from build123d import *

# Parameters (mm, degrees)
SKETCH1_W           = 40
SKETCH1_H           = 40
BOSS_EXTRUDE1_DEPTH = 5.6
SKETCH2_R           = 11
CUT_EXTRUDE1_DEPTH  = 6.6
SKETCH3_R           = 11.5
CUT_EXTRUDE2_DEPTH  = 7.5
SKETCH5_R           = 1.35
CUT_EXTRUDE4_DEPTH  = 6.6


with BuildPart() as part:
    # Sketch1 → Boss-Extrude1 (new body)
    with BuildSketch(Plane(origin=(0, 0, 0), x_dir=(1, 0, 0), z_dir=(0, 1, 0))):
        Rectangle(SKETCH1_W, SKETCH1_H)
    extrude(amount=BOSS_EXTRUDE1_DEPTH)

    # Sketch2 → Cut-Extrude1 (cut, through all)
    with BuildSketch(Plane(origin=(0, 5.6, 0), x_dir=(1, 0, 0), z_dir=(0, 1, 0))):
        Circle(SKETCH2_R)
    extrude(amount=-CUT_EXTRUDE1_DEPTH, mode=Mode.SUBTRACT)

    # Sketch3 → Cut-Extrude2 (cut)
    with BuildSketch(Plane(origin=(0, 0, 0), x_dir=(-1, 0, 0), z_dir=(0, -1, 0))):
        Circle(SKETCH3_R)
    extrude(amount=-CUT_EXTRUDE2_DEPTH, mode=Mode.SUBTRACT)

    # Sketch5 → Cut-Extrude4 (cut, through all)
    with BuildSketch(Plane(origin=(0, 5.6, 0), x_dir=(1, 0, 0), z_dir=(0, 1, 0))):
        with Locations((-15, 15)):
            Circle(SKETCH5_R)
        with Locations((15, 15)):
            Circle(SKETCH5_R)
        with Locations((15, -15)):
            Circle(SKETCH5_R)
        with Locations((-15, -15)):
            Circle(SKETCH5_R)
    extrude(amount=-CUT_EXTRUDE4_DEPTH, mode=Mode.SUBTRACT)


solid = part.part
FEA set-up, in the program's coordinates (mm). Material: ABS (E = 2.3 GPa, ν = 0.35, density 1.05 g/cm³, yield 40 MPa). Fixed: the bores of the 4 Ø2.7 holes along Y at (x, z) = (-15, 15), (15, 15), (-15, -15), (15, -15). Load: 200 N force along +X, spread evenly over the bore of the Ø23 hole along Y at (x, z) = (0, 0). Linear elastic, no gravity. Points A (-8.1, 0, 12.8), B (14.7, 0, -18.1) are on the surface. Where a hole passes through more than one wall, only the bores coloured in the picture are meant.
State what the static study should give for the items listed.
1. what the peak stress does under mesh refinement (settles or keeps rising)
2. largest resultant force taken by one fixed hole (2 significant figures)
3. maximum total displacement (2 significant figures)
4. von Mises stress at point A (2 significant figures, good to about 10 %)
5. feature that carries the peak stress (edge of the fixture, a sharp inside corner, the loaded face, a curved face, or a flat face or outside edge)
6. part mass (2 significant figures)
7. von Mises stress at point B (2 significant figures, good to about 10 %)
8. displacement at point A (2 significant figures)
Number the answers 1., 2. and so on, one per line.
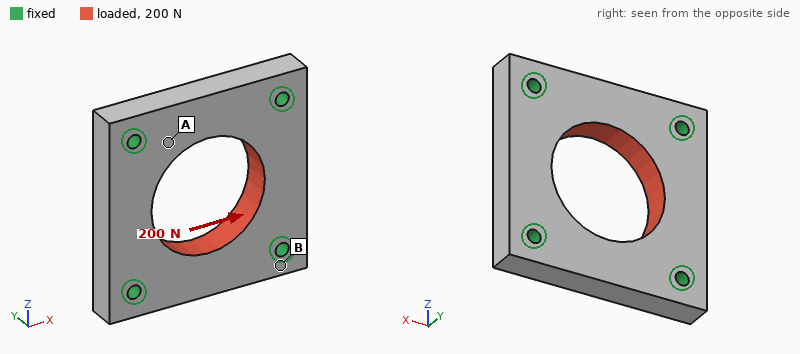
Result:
1. keeps rising
2. 51 N
3. 12 µm
4. 0.84 MPa
5. edge of the fixture
6. 6.8 g
7. 0.41 MPa
8. 3.5 µm
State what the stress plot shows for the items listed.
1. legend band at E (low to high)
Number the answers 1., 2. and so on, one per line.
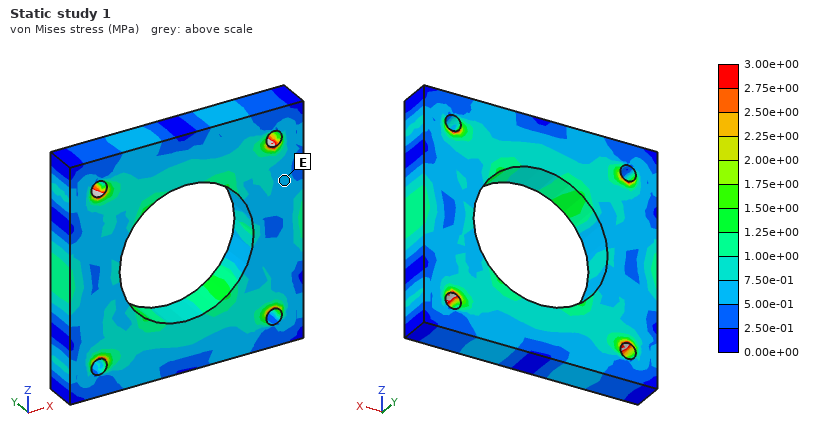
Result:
1. 5.00e-01 to 7.50e-01 MPa
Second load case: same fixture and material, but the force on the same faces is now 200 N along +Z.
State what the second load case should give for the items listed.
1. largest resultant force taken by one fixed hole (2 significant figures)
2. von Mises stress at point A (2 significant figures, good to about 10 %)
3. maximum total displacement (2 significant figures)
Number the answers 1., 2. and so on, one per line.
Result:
1. 51 N
2. 0.77 MPa
3. 12 µm
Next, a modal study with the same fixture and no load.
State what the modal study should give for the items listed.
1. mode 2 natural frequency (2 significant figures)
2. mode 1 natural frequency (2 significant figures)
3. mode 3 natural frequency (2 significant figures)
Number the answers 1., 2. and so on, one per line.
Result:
1. 7700 Hz
2. 7600 Hz
3. 8000 Hz
